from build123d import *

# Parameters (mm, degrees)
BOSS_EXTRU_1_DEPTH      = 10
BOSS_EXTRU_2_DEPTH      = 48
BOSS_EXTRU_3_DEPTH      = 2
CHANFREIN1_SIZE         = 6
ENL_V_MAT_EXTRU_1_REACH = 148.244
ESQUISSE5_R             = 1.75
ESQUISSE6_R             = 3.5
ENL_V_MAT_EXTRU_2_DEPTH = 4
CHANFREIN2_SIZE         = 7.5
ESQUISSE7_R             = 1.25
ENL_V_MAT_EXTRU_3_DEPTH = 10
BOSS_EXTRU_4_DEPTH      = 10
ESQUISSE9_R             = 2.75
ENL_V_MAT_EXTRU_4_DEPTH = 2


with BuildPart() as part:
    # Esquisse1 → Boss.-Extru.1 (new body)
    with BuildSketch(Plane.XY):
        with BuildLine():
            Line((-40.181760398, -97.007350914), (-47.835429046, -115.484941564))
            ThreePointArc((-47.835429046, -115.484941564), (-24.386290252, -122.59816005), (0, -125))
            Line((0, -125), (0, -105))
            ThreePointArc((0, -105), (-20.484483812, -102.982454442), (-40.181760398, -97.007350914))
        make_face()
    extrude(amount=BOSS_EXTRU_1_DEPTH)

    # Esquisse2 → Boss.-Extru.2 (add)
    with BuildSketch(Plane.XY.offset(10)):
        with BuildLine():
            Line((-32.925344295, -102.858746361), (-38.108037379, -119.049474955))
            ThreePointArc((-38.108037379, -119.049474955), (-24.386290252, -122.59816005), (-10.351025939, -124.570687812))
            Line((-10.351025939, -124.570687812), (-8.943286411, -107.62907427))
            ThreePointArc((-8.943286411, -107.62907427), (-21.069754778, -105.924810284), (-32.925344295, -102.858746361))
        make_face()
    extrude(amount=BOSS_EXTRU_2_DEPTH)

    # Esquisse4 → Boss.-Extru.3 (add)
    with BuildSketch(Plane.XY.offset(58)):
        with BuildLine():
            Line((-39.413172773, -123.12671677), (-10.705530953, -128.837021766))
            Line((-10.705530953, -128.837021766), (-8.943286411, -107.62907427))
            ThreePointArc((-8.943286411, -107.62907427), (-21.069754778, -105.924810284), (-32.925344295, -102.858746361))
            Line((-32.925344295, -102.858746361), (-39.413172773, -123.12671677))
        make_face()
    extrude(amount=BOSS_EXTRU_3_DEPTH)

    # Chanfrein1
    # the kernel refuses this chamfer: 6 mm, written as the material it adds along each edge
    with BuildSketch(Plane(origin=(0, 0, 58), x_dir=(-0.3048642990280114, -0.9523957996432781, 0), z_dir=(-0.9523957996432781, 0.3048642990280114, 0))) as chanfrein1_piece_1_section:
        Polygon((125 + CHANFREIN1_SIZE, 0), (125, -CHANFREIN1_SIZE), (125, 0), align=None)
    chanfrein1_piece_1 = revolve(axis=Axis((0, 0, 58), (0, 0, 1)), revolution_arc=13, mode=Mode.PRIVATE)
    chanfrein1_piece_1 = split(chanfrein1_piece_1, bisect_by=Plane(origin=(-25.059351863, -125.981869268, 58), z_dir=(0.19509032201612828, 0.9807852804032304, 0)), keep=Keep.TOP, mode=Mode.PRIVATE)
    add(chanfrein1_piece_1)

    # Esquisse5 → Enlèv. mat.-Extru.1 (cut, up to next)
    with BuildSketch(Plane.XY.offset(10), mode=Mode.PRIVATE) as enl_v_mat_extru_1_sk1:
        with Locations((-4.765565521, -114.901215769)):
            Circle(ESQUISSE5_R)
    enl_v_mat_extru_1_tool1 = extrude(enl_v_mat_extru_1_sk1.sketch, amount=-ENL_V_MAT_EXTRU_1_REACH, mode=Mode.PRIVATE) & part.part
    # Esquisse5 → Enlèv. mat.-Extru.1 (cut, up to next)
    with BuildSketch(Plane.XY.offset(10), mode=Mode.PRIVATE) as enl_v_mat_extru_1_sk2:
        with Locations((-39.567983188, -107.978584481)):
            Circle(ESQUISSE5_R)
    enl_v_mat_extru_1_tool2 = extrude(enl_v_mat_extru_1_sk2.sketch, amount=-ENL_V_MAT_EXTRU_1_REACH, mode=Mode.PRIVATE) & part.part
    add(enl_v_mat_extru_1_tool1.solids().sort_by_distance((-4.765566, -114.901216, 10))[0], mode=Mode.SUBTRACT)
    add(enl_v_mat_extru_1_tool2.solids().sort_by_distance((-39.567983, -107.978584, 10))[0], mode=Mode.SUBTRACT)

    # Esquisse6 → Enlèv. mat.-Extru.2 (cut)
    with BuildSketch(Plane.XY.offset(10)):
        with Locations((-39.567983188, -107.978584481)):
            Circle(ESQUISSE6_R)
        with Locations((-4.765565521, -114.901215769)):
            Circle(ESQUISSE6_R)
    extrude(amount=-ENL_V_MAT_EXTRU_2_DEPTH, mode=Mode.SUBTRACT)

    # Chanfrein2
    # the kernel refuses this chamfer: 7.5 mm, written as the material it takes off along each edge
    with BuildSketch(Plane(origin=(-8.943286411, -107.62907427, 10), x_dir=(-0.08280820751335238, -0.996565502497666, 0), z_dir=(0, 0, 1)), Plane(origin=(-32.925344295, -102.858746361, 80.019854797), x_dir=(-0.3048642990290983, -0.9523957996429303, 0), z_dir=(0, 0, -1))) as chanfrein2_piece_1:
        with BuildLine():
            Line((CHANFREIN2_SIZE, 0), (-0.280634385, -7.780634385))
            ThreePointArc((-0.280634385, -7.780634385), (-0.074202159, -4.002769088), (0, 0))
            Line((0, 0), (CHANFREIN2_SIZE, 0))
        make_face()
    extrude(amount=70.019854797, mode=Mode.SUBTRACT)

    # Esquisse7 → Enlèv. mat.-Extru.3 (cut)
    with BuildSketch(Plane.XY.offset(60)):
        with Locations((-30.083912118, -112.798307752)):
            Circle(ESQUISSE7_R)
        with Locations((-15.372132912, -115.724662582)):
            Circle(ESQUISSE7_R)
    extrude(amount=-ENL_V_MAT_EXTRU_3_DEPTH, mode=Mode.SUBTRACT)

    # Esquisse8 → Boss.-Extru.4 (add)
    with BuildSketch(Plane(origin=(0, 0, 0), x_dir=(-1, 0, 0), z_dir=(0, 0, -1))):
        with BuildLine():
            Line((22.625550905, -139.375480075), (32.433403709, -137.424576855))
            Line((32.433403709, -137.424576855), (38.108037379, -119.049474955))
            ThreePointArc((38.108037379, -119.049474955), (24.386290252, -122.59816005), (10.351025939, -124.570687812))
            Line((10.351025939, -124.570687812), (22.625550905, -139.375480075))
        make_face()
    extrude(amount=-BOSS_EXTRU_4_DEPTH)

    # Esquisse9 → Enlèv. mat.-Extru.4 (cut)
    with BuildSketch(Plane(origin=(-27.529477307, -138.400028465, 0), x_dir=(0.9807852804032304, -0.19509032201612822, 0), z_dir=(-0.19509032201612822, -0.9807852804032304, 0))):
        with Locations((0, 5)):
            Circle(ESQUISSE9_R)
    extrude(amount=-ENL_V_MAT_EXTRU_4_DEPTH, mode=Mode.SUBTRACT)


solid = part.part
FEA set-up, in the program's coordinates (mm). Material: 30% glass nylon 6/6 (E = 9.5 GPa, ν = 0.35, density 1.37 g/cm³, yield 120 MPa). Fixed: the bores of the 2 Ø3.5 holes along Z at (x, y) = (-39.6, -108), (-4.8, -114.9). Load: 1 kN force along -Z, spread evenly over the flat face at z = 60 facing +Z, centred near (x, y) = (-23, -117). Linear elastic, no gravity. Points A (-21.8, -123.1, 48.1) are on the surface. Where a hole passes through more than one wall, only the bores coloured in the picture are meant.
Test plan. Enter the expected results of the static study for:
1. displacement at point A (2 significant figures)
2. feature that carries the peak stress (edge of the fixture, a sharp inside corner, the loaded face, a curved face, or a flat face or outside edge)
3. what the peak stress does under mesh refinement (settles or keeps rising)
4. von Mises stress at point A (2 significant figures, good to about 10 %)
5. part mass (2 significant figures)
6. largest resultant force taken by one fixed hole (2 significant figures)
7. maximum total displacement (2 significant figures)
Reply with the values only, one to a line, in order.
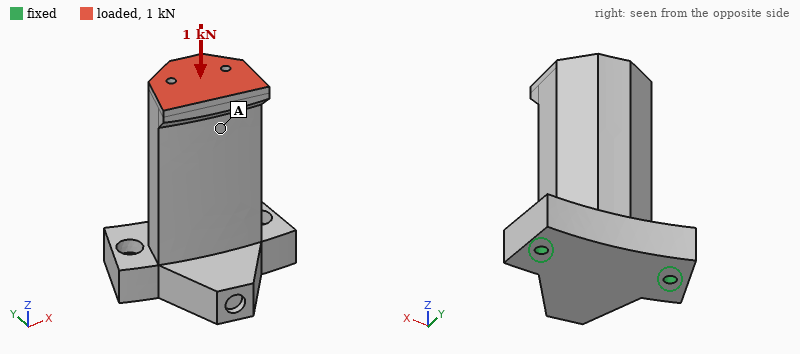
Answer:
0.19 mm
edge of the fixture
keeps rising
4.9 MPa
44 g
540 N
0.25 mm
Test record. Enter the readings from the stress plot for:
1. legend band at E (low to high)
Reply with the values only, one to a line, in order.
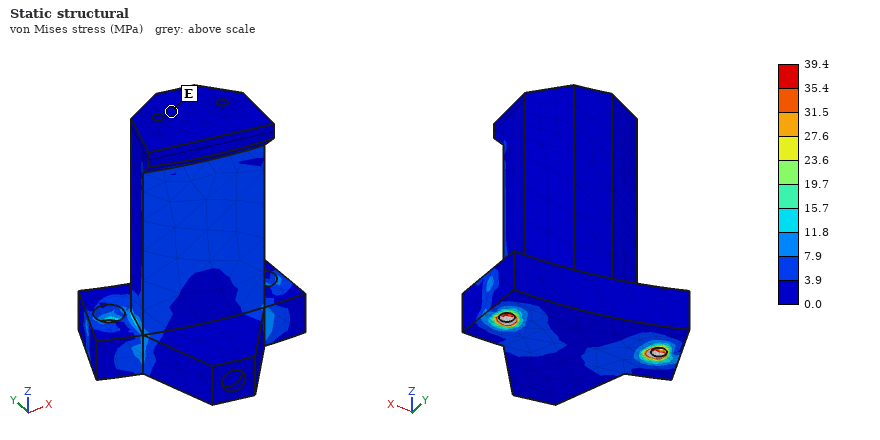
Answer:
0.0 to 3.9 MPa
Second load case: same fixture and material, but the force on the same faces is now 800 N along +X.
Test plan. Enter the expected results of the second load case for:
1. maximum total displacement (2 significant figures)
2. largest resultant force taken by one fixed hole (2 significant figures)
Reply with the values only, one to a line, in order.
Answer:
0.62 mm
1.4 kN
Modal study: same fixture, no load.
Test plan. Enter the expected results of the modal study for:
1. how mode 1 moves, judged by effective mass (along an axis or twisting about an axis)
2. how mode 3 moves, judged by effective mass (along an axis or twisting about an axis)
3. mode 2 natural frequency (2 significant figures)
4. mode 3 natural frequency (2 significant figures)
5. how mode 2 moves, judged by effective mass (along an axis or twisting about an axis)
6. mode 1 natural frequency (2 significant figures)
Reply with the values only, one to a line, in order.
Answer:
along Y
along Z
2400 Hz
5100 Hz
along X
910 Hz
